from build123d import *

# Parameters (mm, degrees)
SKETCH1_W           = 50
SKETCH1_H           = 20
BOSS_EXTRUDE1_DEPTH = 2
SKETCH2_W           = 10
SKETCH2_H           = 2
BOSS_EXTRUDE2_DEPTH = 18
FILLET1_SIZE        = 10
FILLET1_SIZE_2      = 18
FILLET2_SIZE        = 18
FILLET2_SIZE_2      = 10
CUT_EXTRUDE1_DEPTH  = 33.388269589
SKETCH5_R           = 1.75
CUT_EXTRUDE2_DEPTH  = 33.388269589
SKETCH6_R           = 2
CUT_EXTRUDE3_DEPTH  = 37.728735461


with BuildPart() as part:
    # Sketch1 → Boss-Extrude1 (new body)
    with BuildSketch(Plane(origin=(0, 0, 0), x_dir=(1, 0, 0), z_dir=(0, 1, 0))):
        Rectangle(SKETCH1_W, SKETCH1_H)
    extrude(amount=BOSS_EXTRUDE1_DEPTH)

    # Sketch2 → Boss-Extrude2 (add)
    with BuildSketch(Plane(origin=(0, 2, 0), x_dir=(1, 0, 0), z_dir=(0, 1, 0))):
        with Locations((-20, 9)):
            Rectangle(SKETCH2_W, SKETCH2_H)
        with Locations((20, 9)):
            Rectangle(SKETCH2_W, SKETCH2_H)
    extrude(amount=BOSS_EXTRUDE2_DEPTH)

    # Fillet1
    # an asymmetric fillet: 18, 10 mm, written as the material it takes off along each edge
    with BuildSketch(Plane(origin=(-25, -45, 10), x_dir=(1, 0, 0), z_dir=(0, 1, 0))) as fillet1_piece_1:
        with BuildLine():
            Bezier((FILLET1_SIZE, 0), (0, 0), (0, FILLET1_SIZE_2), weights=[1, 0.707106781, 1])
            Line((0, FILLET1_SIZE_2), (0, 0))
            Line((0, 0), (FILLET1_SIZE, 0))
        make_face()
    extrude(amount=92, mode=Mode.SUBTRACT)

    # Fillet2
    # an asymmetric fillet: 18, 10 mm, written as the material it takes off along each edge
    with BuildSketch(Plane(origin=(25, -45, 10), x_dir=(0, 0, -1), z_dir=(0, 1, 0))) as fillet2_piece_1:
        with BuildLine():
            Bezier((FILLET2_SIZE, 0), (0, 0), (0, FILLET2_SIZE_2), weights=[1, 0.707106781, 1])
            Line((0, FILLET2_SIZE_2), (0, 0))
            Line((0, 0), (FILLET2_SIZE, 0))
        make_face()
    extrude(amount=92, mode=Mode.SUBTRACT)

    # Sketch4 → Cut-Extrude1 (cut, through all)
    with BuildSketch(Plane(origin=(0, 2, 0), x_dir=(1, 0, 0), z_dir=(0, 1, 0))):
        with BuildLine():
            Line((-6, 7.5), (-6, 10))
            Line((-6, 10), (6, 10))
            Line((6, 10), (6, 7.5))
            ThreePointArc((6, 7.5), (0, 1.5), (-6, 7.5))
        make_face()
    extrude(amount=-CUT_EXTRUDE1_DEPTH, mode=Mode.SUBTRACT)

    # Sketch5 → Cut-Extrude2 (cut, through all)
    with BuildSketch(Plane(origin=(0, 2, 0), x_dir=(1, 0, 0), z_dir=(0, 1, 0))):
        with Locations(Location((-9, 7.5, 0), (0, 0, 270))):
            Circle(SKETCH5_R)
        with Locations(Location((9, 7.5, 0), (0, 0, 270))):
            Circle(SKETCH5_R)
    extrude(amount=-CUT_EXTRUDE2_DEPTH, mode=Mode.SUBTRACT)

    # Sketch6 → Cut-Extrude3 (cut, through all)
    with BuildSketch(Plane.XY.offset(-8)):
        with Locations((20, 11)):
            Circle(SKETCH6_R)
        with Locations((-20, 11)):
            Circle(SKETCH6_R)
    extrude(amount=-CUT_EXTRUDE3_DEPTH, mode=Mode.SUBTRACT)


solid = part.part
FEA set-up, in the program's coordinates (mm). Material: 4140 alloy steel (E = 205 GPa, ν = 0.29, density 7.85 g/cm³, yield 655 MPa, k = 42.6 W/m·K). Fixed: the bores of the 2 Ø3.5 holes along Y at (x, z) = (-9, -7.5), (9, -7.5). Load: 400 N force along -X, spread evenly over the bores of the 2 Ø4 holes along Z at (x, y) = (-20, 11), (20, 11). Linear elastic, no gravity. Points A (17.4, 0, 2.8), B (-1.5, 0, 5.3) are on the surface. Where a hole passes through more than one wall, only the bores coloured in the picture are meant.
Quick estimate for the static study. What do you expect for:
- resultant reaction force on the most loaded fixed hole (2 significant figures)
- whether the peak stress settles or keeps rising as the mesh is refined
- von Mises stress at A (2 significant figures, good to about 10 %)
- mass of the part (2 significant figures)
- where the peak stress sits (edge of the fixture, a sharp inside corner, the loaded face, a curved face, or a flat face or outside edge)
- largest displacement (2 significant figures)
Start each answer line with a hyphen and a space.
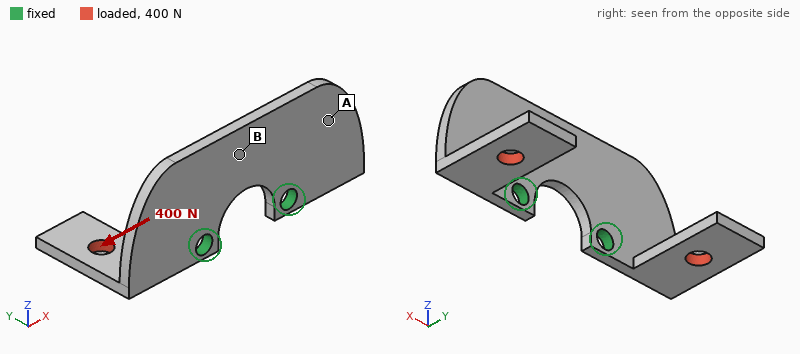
- 210 N
- keeps rising
- 90 MPa
- 18 g
- edge of the fixture
- 0.21 mm
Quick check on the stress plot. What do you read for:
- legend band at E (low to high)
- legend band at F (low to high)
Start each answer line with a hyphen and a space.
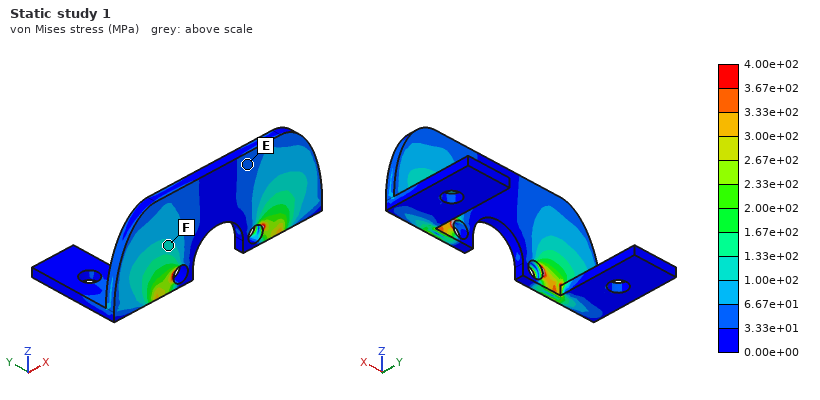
- 3.33e+01 to 6.67e+01 MPa
- 1.00e+02 to 1.33e+02 MPa
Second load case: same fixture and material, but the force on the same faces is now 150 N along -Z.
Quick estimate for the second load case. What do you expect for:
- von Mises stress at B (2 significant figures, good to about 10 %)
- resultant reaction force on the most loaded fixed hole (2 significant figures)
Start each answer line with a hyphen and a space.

- 15 MPa
- 92 N
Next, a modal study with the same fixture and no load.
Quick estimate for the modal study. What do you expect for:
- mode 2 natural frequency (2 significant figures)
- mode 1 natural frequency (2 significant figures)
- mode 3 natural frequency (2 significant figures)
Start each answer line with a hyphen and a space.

- 3000 Hz
- 2800 Hz
- 3100 Hz
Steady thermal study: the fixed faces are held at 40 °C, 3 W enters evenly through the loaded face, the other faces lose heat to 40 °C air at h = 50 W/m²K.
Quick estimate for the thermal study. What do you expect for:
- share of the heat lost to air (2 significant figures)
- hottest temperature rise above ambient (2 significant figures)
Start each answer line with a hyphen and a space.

- 42 %
- 26 K
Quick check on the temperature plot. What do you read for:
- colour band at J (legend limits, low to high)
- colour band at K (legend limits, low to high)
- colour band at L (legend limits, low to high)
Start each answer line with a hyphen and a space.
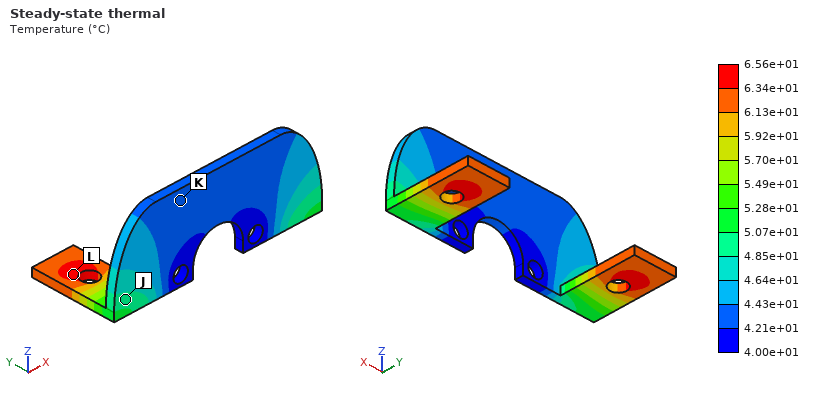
- 4.85e+01 to 5.07e+01 °C
- 4.21e+01 to 4.43e+01 °C
- 6.34e+01 to 6.56e+01 °C
